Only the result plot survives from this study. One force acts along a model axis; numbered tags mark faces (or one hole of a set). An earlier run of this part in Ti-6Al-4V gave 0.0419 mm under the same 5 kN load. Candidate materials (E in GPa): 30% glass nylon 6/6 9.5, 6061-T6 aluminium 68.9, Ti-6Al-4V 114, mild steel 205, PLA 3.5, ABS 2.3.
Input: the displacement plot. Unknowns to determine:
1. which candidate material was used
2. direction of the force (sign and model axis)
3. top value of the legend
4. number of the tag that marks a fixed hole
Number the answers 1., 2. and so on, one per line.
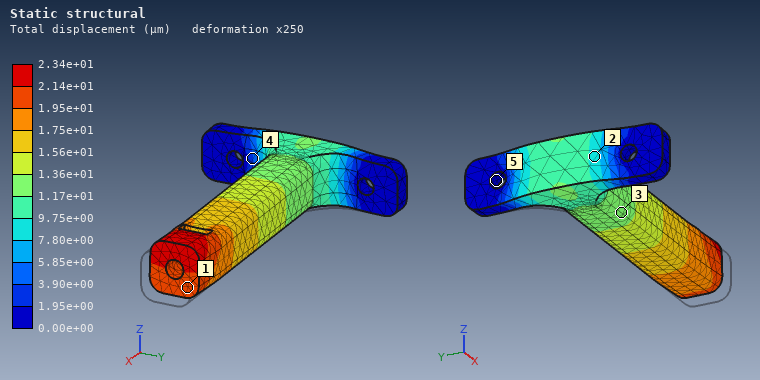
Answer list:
1. mild steel
2. -X
3. 2.34e+01 µm
4. 5
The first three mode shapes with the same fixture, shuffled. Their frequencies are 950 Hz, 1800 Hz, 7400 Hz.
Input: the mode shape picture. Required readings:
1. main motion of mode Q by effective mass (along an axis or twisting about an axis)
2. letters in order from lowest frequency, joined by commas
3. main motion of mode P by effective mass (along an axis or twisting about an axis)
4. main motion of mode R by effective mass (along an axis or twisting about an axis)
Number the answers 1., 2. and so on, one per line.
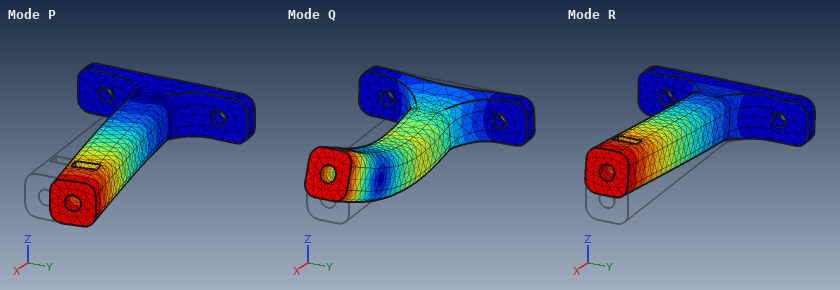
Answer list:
1. along Z
2. R, P, Q
3. along Y
4. along Z
